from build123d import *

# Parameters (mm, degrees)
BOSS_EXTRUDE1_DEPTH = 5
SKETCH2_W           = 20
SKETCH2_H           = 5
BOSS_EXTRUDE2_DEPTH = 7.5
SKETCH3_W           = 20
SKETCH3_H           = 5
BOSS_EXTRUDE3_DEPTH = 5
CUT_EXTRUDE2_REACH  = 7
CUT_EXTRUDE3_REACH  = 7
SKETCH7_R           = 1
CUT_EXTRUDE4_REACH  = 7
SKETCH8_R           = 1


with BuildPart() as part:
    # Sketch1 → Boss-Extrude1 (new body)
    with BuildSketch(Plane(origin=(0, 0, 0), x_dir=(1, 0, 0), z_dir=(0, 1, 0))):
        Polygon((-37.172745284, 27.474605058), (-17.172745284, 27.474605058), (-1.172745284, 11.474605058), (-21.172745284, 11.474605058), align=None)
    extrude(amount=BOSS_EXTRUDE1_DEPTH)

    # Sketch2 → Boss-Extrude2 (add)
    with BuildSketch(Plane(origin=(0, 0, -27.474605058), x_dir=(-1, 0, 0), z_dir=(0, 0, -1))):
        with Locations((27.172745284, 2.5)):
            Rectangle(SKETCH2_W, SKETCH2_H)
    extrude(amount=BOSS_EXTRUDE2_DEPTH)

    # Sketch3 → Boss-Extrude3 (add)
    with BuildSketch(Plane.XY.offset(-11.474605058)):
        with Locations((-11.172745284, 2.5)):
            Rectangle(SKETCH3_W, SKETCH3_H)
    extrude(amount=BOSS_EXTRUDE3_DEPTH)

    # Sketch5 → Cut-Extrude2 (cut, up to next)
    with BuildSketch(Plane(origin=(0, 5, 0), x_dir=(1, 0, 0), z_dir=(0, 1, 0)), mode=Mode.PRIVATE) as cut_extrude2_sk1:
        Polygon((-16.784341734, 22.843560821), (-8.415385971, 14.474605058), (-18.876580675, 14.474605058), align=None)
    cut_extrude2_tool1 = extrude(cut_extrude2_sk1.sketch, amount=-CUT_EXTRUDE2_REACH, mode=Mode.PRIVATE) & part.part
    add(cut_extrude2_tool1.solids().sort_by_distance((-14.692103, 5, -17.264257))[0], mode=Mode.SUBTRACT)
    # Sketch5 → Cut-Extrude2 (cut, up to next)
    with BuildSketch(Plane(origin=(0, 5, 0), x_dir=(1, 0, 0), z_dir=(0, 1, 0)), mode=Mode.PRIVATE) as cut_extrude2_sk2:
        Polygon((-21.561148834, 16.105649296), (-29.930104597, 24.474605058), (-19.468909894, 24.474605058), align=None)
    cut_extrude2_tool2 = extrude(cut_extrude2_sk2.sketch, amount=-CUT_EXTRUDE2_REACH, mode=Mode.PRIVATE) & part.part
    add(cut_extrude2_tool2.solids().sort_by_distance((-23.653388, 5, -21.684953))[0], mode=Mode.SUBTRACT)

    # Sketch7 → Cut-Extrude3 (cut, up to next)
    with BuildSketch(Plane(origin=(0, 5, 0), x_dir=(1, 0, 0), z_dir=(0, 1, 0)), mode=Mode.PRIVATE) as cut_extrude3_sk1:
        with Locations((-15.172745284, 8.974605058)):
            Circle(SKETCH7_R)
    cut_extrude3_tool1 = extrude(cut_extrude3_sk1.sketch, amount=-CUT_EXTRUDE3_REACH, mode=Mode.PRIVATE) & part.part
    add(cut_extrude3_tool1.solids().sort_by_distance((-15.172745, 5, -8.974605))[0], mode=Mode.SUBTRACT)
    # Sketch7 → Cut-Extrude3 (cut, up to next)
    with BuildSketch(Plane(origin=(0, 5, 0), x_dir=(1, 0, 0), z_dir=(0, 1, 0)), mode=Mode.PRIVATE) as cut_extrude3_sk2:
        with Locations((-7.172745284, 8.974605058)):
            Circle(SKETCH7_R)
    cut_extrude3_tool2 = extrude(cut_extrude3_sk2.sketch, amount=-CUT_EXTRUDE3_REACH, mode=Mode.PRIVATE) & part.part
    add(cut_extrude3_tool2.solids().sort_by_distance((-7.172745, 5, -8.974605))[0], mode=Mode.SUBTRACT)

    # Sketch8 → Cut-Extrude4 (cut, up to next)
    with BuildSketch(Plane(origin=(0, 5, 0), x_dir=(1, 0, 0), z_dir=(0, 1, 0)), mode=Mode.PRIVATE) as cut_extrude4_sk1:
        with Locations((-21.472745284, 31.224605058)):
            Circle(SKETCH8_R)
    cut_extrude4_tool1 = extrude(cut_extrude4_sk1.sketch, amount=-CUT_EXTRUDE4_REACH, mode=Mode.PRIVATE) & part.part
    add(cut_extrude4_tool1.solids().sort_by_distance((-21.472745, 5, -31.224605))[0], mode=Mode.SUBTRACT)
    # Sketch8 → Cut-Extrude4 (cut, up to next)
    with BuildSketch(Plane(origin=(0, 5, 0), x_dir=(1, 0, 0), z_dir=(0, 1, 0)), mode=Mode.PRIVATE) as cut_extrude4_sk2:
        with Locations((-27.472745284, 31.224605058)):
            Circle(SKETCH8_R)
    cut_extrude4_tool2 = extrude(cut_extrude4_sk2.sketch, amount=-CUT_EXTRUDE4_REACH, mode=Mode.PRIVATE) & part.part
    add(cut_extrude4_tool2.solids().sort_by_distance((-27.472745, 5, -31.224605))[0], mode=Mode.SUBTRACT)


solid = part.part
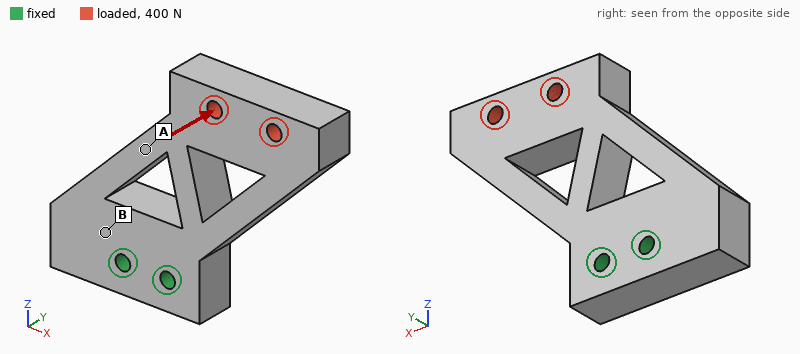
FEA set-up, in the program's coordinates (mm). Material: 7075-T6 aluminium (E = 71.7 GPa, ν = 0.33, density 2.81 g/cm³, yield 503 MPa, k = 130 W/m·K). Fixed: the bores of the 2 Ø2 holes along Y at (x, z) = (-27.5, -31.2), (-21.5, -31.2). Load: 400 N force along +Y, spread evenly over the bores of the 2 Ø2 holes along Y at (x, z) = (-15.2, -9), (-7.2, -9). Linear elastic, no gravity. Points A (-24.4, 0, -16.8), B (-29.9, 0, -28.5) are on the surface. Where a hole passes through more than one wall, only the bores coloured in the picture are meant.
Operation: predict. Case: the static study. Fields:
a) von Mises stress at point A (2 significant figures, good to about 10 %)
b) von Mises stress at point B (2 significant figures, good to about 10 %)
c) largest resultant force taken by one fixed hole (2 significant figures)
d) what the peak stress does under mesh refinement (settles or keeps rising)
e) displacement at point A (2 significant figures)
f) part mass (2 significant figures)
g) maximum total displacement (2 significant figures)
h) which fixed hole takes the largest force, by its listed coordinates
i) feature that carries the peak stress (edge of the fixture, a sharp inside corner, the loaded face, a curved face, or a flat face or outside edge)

150 MPa
58 MPa
550 N
keeps rising
0.11 mm
6.6 g
0.49 mm
(-21.5, -31.2)
edge of the fixture
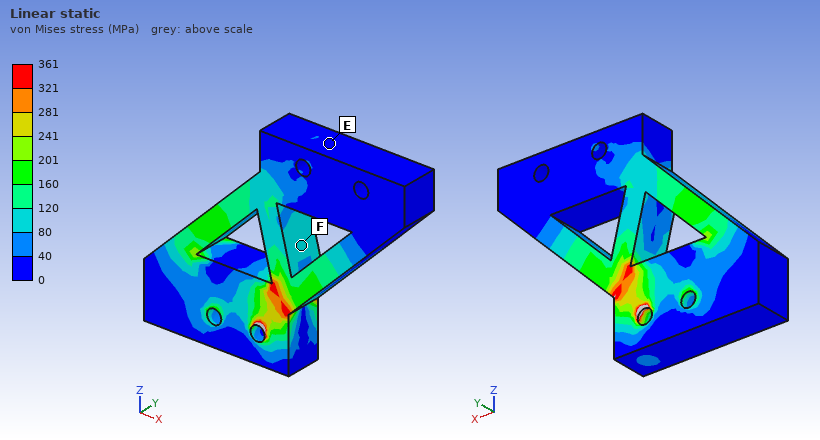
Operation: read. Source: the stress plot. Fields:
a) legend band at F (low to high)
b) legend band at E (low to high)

80 to 120 MPa
0 to 40 MPa
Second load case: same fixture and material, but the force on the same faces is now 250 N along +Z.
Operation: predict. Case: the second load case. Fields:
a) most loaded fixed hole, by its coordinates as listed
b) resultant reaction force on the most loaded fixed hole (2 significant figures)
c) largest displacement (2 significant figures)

(-21.5, -31.2)
560 N
27 µm
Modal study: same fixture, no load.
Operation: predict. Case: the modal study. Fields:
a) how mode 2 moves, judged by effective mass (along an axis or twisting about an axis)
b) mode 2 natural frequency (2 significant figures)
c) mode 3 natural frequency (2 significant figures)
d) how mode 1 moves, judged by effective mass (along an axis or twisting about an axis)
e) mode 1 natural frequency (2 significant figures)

along X
8400 Hz
10 kHz
along Y
3700 Hz
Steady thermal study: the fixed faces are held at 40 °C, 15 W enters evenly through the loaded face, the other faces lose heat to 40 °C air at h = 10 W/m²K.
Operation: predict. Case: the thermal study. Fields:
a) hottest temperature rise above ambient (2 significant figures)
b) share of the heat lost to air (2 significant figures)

68 K
3.6 %
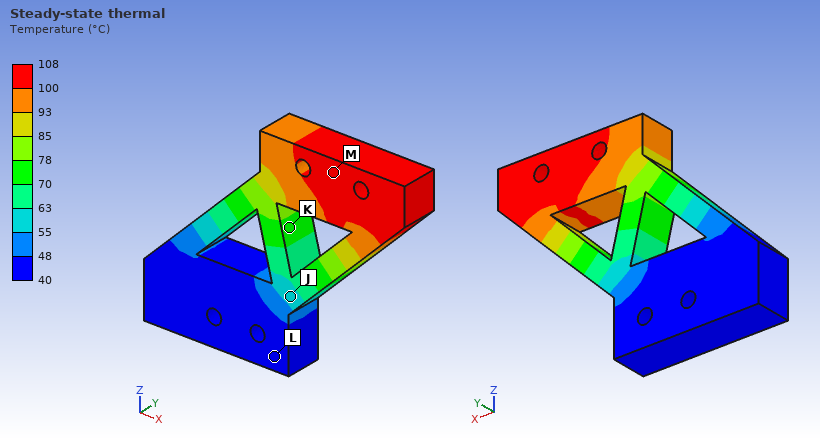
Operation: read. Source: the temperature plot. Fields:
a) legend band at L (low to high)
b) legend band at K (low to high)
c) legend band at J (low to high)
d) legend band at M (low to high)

40 to 48 °C
70 to 78 °C
55 to 63 °C
100 to 108 °C
